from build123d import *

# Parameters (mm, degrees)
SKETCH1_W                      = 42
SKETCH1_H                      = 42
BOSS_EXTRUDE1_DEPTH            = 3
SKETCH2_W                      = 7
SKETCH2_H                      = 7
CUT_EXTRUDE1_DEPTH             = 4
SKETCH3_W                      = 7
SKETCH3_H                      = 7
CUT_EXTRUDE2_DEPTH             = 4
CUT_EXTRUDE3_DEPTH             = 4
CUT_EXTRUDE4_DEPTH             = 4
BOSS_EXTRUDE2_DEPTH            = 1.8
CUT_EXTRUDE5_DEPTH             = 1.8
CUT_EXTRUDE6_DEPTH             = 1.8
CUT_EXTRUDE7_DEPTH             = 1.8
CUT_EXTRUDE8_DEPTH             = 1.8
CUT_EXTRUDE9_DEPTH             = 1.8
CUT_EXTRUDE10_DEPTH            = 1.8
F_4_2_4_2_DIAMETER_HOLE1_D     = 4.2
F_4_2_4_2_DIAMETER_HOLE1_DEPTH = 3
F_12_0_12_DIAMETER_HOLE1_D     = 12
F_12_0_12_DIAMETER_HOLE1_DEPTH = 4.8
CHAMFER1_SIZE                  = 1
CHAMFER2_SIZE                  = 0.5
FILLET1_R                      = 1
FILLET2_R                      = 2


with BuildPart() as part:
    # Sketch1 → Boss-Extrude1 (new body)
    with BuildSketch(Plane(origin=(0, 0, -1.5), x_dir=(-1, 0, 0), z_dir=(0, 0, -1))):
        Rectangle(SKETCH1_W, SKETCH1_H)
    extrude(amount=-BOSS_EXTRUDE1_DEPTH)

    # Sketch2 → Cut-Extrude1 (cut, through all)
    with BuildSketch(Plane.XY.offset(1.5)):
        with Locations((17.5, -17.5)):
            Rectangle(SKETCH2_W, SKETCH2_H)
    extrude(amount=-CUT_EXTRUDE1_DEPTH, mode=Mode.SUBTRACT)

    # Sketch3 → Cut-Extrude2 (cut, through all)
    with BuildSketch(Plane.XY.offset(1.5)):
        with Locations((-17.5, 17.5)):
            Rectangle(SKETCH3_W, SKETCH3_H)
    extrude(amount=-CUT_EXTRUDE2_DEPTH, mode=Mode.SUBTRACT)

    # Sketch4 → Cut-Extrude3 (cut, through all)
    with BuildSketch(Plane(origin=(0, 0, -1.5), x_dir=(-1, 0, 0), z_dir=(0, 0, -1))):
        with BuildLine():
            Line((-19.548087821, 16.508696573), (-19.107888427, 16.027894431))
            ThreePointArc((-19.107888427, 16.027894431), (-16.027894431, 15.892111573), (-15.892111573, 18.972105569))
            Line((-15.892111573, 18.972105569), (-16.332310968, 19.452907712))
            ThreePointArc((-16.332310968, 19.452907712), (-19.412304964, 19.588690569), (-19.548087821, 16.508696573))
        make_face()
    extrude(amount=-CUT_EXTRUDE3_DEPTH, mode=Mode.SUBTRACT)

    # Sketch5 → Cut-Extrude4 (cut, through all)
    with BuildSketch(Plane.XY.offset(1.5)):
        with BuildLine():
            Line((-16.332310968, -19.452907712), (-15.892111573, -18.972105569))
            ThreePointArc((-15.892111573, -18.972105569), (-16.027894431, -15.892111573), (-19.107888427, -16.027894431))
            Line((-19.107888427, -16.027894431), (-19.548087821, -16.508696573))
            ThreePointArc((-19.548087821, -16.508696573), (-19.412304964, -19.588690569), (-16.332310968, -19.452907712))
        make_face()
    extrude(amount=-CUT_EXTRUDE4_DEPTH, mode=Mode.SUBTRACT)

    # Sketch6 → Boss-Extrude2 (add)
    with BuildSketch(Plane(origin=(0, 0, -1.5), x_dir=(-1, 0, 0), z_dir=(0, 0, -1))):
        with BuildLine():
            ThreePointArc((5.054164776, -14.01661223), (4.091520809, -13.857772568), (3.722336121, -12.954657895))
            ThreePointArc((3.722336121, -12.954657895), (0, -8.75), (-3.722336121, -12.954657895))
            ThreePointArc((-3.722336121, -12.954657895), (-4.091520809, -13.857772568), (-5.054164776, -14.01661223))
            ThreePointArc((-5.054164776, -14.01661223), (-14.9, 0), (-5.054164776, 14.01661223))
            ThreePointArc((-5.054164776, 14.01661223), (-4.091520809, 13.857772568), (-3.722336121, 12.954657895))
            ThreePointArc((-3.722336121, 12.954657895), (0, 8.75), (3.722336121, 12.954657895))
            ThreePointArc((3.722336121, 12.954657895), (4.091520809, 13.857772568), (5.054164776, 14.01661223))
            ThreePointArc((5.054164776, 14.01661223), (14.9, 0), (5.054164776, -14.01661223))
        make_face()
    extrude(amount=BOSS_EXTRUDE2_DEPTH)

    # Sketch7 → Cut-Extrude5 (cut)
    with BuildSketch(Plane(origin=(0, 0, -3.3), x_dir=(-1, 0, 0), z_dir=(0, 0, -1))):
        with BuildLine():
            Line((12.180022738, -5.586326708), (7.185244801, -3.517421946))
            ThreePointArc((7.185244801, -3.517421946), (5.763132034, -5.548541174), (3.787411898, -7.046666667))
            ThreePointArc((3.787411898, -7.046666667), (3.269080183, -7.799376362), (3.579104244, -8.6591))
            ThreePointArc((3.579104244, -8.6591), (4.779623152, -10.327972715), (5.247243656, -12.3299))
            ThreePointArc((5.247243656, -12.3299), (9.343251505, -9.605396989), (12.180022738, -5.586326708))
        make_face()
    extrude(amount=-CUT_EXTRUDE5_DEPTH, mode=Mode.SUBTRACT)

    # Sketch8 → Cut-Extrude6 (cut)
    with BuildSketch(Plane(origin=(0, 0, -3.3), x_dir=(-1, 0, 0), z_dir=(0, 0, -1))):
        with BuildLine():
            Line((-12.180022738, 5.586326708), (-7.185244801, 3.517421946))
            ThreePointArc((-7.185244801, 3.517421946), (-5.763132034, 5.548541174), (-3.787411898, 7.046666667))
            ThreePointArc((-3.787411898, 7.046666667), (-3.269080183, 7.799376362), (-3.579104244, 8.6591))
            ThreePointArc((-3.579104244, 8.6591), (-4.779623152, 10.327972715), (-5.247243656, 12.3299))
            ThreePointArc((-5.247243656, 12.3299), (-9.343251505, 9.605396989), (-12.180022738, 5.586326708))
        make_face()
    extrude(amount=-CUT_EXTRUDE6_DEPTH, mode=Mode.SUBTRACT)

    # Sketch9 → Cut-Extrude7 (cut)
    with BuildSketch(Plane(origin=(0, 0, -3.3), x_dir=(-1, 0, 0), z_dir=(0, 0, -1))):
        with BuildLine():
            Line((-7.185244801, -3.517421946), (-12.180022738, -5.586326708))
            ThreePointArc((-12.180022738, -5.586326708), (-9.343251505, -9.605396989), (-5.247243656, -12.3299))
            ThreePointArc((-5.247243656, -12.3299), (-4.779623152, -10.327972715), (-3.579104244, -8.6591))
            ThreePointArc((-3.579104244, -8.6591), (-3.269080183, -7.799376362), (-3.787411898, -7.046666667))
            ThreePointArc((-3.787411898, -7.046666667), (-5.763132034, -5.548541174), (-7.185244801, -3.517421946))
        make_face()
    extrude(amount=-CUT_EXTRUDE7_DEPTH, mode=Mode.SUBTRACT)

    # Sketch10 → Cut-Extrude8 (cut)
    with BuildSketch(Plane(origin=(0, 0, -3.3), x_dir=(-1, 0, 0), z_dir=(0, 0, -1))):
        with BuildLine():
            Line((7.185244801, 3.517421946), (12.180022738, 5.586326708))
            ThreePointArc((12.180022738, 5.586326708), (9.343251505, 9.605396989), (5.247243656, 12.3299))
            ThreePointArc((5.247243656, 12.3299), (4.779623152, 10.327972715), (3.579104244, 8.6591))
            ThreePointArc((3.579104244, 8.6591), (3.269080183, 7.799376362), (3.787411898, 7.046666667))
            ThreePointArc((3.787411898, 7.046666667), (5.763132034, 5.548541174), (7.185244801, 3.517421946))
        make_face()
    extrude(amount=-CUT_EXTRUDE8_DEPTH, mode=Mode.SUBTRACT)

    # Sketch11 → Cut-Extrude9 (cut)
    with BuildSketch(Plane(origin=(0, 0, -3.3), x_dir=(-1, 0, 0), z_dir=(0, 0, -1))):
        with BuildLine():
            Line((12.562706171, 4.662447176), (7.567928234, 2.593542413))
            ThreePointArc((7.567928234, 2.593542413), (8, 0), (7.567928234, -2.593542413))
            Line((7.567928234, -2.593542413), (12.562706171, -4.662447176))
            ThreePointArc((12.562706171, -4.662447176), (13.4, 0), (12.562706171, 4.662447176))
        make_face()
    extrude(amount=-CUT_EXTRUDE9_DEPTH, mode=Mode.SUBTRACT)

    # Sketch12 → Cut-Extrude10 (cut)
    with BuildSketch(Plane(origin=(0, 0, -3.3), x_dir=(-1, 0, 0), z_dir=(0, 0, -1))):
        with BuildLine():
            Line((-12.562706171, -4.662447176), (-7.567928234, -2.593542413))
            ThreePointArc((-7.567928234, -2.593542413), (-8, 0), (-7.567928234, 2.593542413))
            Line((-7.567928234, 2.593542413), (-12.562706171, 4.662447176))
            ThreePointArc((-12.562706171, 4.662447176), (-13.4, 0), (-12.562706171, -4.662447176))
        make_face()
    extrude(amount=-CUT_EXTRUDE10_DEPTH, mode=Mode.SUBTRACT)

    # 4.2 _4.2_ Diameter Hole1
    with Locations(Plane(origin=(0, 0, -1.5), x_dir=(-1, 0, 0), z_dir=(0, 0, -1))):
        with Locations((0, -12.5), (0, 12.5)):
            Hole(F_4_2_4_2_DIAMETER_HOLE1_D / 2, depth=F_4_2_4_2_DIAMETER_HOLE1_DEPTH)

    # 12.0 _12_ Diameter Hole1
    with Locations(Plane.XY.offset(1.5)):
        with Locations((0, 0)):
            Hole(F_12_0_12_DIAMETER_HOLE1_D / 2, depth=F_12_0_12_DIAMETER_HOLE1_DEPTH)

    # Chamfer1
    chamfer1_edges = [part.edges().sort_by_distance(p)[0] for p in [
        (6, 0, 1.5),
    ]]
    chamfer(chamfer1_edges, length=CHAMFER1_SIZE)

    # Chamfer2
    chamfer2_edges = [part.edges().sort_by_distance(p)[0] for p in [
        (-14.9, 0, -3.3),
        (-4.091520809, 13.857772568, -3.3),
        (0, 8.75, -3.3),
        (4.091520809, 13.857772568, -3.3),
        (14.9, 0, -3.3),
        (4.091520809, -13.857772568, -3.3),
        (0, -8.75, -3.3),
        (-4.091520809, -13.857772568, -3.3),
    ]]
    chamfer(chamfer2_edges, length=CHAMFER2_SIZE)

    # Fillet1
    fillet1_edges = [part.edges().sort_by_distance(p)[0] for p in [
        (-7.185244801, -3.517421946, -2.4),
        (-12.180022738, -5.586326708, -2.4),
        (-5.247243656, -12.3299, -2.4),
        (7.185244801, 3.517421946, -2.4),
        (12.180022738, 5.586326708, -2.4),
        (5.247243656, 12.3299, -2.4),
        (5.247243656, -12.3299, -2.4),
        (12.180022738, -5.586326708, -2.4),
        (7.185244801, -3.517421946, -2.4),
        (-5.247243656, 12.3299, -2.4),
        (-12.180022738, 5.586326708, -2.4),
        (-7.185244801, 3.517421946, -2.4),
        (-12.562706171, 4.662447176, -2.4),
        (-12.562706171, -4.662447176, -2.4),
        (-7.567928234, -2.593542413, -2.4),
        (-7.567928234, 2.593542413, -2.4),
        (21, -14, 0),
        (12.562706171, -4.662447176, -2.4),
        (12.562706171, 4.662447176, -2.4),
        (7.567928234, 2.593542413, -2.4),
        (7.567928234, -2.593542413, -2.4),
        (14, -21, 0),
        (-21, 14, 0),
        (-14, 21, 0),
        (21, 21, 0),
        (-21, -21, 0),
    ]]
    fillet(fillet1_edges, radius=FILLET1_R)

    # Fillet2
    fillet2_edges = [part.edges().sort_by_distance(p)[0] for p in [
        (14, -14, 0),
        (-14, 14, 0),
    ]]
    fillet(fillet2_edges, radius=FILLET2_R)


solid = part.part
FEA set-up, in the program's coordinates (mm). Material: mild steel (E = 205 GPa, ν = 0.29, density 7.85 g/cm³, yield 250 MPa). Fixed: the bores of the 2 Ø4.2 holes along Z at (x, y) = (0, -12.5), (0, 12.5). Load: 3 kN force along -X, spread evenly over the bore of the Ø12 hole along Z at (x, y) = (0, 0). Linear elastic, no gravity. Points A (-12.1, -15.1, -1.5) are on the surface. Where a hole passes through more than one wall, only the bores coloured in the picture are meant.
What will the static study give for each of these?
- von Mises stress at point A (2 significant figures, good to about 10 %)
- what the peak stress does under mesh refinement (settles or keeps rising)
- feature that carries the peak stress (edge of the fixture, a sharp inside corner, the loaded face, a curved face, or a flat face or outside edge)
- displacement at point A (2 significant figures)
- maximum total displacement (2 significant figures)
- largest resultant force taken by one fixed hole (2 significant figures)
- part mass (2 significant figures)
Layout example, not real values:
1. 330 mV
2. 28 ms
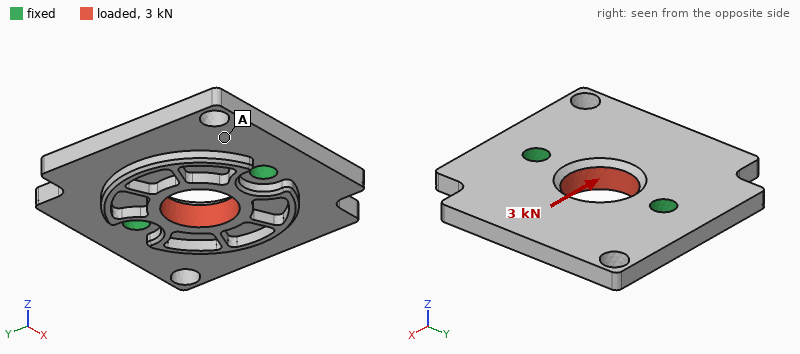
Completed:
1. 11 MPa
2. keeps rising
3. edge of the fixture
4. 4.9 µm
5. 12 µm
6. 1.5 kN
7. 39 g
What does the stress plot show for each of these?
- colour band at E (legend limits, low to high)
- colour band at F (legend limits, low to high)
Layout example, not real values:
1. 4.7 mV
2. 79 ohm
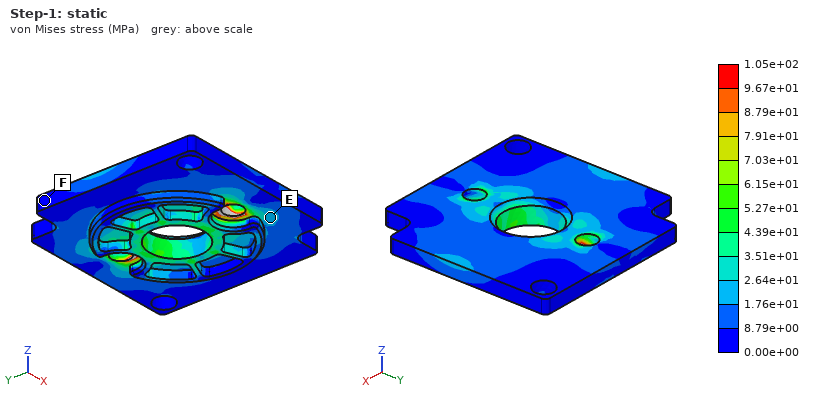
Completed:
1. 1.76e+01 to 2.64e+01 MPa
2. 0.00e+00 to 8.79e+00 MPa
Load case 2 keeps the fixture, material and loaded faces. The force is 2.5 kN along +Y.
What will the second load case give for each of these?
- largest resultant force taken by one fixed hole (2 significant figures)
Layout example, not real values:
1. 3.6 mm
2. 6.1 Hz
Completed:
1. 1.3 kN
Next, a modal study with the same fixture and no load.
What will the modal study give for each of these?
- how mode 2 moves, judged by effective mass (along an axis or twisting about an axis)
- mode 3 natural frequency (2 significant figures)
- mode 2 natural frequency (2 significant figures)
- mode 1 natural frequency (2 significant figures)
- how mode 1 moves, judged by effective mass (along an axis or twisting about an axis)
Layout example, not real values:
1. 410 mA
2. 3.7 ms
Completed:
1. along Z
2. 11 kHz
3. 6800 Hz
4. 5900 Hz
5. twisting about Y
